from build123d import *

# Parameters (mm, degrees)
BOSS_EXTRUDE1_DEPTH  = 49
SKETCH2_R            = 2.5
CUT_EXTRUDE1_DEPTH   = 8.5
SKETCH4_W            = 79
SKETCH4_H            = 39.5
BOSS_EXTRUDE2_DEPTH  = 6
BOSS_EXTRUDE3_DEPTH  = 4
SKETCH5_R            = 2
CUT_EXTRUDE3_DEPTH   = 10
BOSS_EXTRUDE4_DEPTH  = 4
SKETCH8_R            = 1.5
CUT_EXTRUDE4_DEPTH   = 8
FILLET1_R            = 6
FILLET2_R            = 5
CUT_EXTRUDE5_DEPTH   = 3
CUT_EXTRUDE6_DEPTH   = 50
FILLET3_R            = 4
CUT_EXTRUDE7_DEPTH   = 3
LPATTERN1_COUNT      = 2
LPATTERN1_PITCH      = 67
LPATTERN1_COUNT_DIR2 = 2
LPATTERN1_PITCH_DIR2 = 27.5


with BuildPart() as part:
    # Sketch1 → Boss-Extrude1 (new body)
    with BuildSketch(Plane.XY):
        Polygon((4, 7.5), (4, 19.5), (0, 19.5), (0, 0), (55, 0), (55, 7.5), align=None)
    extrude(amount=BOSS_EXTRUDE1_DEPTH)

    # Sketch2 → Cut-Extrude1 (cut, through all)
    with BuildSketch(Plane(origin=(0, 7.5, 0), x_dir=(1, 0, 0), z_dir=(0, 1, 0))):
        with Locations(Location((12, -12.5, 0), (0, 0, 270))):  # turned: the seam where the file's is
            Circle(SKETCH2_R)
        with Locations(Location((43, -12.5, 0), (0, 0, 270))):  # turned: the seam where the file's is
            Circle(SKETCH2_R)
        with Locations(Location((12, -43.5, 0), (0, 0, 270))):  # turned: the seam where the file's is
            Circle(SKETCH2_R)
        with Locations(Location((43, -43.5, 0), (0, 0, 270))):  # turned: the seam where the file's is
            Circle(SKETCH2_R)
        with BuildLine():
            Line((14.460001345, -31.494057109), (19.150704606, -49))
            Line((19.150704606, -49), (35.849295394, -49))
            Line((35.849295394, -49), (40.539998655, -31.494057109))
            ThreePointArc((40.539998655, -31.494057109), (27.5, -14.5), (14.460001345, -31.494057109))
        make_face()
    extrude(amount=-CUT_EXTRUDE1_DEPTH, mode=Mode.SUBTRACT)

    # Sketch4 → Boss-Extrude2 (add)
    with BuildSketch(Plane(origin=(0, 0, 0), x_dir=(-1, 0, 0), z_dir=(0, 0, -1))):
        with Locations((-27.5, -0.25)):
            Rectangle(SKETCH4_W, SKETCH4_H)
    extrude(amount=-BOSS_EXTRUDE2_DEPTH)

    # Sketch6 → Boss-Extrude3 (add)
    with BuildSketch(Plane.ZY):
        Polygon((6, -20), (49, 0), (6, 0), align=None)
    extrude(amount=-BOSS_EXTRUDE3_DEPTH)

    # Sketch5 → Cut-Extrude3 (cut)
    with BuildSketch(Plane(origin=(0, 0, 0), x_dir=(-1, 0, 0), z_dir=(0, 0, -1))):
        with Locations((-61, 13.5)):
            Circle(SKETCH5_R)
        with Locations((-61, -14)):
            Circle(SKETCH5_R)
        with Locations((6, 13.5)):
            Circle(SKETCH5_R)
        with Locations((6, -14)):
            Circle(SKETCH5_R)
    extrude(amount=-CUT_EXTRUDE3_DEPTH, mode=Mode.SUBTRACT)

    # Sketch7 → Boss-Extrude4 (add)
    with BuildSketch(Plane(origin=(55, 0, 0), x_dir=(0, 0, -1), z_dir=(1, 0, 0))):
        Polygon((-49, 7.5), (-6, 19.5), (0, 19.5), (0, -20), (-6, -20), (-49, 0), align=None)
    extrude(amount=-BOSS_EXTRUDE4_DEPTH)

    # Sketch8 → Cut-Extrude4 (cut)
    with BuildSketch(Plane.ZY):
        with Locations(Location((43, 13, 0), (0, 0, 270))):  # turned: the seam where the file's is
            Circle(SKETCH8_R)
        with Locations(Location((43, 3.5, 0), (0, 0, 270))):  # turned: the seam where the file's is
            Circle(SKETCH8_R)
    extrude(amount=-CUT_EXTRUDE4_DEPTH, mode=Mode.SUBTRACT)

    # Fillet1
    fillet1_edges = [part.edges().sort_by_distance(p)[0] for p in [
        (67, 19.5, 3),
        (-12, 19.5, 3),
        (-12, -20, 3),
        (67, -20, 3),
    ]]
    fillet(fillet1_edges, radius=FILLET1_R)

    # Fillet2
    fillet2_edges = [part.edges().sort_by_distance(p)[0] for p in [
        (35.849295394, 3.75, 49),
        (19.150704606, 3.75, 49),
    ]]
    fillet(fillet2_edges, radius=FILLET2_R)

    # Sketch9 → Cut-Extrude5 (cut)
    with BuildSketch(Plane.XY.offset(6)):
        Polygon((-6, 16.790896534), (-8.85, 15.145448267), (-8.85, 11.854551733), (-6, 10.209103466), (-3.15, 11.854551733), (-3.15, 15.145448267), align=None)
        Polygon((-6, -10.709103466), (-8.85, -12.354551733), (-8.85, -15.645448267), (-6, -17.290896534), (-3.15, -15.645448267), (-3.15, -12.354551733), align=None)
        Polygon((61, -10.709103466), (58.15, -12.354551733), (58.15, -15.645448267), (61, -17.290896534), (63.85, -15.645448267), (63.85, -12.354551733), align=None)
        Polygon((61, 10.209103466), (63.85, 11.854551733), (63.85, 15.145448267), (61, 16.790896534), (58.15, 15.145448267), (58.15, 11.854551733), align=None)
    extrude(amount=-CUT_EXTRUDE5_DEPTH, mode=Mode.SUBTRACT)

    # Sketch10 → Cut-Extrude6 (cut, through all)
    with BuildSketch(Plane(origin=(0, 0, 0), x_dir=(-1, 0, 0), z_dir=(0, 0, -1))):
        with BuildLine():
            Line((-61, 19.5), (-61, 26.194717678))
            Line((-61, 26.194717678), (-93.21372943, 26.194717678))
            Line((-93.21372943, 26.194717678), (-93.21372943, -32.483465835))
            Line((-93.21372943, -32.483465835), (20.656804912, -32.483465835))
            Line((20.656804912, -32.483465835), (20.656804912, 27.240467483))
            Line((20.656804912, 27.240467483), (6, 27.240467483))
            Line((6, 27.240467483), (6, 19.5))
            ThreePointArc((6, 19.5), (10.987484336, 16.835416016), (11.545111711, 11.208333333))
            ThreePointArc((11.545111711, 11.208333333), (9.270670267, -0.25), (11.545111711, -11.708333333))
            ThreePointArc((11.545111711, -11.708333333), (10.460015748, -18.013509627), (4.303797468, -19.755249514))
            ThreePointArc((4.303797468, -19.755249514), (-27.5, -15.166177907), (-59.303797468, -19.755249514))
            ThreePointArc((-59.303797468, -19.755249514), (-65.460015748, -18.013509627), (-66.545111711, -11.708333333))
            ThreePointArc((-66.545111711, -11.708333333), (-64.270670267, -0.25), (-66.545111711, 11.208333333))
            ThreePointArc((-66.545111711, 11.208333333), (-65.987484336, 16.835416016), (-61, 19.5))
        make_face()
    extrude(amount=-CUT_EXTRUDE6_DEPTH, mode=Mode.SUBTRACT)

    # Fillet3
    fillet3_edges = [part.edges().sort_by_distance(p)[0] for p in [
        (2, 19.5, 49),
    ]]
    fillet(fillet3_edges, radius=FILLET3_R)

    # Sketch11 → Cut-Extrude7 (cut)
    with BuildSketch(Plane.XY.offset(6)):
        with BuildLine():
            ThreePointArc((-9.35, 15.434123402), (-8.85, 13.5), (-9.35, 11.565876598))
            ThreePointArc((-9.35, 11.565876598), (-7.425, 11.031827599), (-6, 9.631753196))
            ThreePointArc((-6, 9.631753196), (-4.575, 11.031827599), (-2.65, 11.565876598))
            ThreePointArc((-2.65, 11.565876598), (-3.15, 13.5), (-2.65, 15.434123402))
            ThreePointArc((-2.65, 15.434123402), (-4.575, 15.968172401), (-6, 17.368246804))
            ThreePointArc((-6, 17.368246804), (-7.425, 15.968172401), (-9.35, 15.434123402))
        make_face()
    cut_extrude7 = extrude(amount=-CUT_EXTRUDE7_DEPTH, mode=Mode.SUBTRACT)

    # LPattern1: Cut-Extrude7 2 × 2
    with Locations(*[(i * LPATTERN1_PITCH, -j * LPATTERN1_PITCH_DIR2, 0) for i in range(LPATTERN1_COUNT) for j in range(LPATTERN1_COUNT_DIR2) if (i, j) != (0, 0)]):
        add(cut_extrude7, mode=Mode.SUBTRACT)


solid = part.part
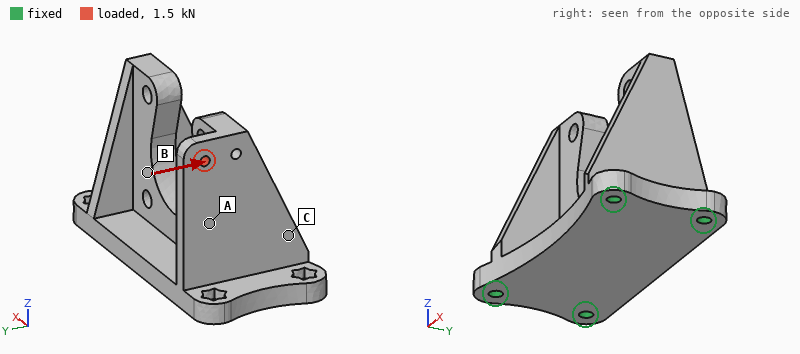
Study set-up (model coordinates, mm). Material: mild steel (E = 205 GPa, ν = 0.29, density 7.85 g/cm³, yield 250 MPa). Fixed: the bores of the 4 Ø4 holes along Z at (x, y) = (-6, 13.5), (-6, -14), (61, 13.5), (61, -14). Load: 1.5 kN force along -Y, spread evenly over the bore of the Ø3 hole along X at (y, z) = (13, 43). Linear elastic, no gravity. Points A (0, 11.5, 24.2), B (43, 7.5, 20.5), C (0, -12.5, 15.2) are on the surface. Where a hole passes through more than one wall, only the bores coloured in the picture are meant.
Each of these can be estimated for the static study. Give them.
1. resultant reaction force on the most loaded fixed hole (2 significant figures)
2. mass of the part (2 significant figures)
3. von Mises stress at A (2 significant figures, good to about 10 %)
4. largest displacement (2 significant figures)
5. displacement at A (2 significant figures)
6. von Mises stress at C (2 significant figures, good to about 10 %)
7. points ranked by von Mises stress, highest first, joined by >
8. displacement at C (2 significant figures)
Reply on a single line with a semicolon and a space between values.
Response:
2.3 kN; 270 g; 25 MPa; 48 µm; 20 µm; 56 MPa; C > A > B; 14 µm
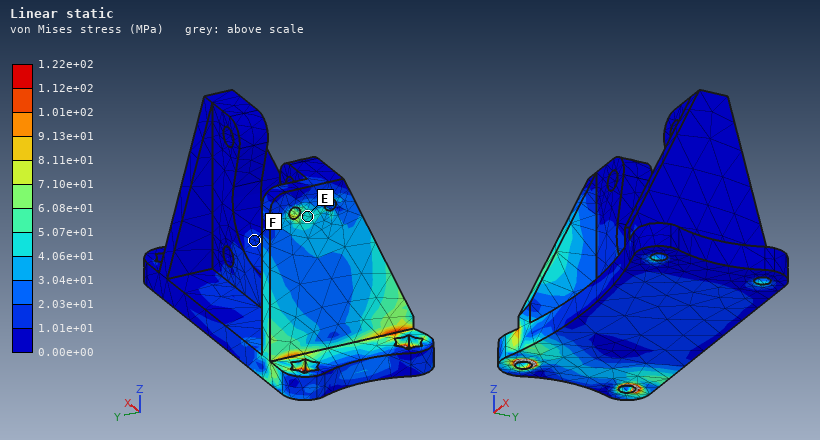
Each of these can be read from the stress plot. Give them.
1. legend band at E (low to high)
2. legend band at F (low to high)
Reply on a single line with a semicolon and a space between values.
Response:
4.06e+01 to 5.07e+01 MPa; 1.01e+01 to 2.03e+01 MPa
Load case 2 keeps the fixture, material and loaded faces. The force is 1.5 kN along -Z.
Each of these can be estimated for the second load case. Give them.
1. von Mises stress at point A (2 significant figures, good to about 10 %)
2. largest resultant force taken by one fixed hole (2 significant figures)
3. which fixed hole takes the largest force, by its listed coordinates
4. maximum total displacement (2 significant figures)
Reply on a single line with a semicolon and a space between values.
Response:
23 MPa; 1.4 kN; (-6, 13.5); 17 µm
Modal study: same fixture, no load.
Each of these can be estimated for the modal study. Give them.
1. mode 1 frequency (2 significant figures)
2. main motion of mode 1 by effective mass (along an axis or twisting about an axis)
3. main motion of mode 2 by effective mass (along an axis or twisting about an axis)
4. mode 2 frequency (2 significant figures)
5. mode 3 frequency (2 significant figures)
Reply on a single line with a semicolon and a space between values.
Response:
4800 Hz; along Z; along Y; 5500 Hz; 6500 Hz
